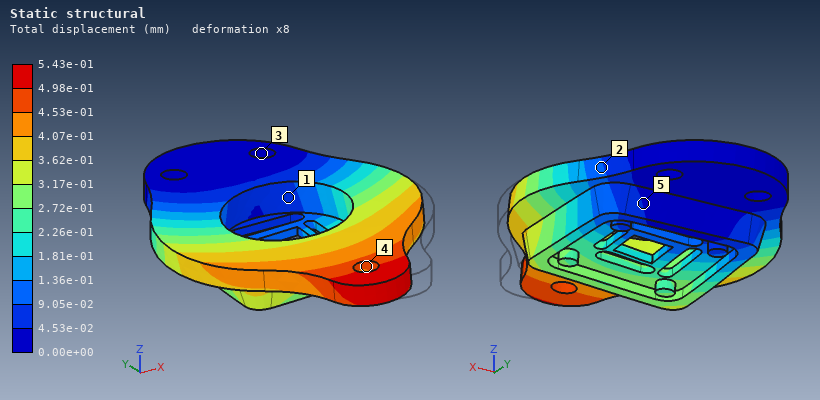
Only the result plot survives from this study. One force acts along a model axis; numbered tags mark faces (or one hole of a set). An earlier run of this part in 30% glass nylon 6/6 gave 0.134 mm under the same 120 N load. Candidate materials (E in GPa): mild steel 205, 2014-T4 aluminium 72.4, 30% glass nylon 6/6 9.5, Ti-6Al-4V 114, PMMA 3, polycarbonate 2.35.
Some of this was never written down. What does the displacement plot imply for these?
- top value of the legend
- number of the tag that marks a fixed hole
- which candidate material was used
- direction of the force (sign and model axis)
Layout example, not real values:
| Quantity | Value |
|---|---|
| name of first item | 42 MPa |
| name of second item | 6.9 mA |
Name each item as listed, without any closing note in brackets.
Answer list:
| Quantity | Value |
|---|---|
| top value of the legend | 5.43e-01 mm |
| number of the tag that marks a fixed hole | 3 |
| which candidate material was used | polycarbonate |
| direction of the force | -X |
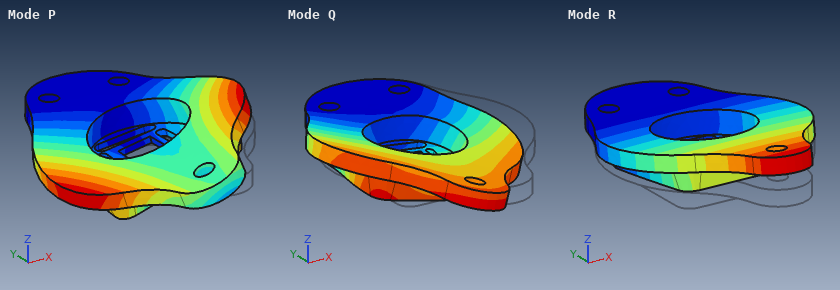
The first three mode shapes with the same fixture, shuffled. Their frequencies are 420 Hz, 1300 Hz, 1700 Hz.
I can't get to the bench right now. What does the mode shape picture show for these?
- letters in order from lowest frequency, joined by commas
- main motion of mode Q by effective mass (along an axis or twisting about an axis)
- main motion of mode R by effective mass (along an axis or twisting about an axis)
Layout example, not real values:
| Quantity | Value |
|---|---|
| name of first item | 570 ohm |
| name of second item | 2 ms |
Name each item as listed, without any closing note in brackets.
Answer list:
| Quantity | Value |
|---|---|
| letters in order from lowest frequency, joined by commas | R, P, Q |
| main motion of mode Q by effective mass | along X |
| main motion of mode R by effective mass | along Z |
